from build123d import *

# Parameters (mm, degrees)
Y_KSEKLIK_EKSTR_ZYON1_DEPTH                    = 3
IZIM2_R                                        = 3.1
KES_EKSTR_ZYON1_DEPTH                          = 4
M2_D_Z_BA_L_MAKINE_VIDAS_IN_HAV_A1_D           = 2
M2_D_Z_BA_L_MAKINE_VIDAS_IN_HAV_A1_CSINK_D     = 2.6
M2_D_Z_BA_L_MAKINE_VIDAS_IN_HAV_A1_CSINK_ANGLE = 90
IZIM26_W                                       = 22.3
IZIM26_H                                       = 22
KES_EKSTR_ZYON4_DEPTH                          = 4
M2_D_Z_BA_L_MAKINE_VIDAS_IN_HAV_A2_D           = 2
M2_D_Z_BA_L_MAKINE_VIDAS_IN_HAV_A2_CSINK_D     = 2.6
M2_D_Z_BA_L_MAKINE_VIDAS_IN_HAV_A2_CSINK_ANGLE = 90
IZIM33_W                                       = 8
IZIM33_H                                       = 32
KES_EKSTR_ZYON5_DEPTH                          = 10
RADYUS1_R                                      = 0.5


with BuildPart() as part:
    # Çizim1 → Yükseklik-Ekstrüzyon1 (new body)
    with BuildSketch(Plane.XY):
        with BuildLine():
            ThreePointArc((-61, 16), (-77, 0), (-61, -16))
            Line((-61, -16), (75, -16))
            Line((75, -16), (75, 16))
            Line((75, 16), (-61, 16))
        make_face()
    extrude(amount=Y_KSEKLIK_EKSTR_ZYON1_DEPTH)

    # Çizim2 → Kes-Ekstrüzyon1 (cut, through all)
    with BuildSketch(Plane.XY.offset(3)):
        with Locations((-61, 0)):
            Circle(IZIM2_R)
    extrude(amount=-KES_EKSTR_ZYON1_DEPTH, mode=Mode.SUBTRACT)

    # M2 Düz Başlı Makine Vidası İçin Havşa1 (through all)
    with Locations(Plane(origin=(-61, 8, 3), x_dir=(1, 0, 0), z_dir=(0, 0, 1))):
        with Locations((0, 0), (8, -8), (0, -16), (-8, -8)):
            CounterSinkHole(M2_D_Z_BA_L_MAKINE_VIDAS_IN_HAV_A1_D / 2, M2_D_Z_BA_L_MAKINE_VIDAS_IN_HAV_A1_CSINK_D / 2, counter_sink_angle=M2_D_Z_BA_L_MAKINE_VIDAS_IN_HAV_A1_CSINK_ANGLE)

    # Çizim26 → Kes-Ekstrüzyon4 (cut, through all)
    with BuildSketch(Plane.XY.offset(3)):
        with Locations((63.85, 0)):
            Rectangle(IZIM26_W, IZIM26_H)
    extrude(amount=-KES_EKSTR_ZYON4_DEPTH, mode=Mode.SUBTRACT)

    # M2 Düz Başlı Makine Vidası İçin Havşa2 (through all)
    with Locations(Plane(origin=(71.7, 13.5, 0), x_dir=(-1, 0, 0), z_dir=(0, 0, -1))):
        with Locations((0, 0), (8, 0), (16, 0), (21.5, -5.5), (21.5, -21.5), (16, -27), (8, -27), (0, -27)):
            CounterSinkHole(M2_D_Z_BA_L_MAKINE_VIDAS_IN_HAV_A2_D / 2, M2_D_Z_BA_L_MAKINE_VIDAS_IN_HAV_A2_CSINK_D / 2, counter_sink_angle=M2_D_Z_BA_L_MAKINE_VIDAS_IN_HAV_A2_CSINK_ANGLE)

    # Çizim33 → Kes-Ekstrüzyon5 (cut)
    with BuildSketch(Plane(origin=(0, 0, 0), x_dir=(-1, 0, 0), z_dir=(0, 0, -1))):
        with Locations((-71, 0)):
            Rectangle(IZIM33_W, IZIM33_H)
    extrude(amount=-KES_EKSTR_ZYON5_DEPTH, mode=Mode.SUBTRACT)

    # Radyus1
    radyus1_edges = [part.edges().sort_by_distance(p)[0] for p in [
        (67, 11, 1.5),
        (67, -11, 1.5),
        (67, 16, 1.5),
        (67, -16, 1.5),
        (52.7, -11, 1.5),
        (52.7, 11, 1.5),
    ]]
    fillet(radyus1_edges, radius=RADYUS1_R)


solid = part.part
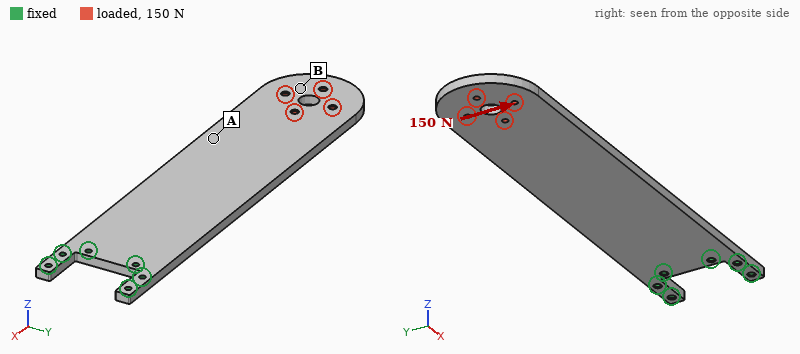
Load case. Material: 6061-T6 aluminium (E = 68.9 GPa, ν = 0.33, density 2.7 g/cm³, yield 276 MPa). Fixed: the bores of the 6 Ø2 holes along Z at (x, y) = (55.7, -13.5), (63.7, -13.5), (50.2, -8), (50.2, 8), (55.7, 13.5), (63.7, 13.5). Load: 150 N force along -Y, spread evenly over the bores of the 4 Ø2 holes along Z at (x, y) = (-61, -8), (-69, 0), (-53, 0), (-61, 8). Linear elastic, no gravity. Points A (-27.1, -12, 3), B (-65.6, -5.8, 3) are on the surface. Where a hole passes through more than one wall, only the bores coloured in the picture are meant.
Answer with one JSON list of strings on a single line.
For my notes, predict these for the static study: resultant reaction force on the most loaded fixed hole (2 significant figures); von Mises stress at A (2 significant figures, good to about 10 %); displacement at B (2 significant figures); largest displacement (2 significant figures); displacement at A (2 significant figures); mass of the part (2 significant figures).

["440 N", "7.6 MPa", "0.15 mm", "0.17 mm", "0.084 mm", "33 g"]
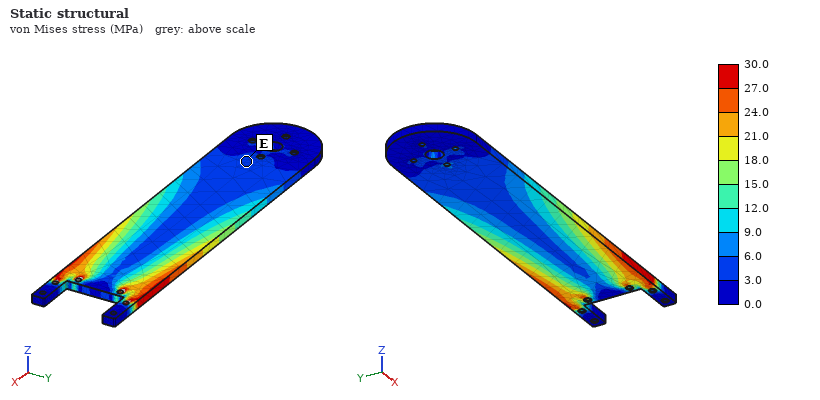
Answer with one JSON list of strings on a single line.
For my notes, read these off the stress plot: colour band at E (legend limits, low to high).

["3.0 to 6.0 MPa"]
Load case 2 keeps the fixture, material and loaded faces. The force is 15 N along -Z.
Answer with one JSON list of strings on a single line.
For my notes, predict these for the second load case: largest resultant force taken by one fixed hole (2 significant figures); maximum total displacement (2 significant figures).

["50 N", "1.7 mm"]
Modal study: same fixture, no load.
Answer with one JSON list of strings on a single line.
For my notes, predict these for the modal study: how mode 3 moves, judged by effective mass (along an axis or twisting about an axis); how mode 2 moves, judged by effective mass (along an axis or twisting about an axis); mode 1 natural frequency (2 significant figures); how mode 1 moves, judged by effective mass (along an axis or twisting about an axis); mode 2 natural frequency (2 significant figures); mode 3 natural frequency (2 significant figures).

["twisting about X", "along Z", "160 Hz", "along Z", "990 Hz", "1200 Hz"]
